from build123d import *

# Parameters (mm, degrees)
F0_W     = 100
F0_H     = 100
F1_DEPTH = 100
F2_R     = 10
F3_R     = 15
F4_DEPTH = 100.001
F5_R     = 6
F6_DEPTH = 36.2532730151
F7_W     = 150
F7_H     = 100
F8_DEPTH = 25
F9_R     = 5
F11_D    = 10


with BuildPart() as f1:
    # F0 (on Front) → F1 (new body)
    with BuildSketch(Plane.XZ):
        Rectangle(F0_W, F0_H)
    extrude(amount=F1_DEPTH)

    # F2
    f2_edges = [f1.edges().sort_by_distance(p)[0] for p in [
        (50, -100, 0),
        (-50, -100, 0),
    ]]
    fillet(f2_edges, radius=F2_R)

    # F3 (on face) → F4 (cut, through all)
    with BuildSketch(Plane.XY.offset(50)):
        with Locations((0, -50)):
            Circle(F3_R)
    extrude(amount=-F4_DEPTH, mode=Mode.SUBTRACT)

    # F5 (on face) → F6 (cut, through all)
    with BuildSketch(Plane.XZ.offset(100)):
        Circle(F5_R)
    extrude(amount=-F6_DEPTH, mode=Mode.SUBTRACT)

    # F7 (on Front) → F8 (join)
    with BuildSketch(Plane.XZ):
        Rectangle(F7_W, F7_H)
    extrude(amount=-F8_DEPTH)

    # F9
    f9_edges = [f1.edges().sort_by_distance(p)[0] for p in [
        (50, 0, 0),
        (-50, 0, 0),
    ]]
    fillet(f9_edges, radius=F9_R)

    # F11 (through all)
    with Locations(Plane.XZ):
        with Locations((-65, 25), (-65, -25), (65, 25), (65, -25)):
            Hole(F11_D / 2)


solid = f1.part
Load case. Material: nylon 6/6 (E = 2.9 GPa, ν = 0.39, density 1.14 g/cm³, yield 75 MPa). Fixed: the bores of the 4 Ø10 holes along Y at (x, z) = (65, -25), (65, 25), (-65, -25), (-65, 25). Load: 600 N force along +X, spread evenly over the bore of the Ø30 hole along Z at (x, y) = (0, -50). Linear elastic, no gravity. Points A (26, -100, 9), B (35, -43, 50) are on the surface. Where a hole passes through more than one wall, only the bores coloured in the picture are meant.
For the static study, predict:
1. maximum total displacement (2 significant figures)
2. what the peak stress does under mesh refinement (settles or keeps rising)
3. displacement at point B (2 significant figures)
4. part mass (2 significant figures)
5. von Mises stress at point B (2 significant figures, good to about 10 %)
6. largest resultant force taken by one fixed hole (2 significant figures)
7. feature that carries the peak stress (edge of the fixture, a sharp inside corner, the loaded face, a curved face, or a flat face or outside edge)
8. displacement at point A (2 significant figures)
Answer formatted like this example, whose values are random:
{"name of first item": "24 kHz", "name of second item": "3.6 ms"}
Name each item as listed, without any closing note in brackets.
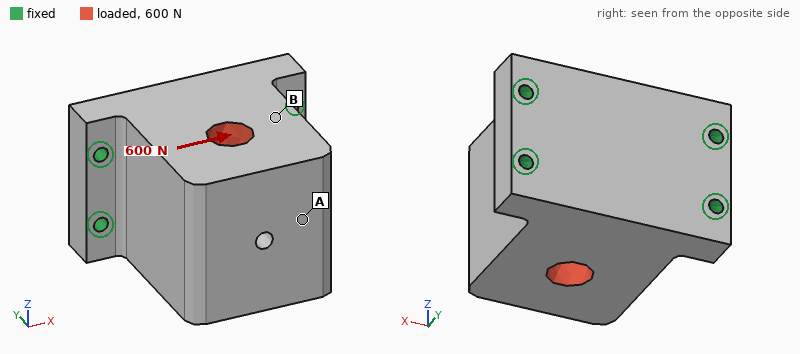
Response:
{"maximum total displacement": "16 µm", "what the peak stress does under mesh refinement": "keeps rising", "displacement at point B": "9.1 µm", "part mass": "1.5 kg", "von Mises stress at point B": "0.13 MPa", "largest resultant force taken by one fixed hole": "220 N", "feature that carries the peak stress": "edge of the fixture", "displacement at point A": "16 µm"}
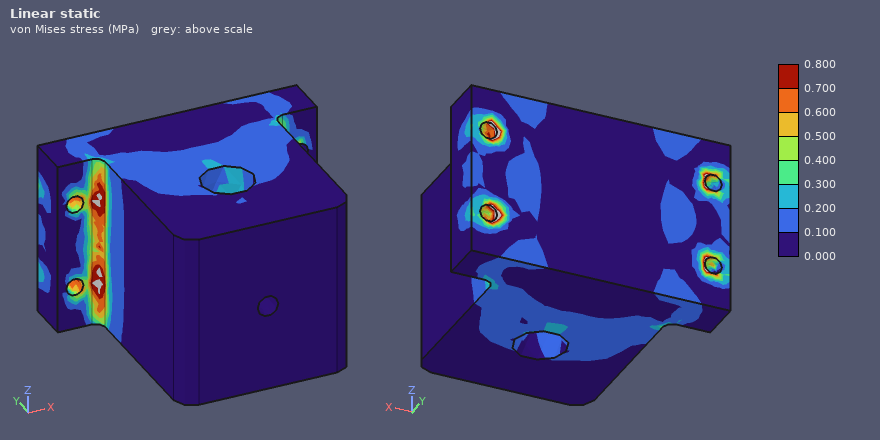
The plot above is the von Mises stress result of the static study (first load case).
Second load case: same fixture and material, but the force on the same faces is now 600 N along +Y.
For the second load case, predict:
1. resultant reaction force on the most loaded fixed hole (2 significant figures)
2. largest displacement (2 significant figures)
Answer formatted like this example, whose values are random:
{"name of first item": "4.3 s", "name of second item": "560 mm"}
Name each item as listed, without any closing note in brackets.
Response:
{"resultant reaction force on the most loaded fixed hole": "160 N", "largest displacement": "7.1 µm"}
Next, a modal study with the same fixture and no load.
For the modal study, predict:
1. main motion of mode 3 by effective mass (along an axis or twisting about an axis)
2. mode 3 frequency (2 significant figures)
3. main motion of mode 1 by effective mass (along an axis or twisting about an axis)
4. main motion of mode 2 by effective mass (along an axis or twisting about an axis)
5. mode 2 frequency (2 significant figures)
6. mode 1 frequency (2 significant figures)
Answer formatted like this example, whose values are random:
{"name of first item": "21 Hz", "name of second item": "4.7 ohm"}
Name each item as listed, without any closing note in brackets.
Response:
{"main motion of mode 3 by effective mass": "along Y", "mode 3 frequency": "1400 Hz", "main motion of mode 1 by effective mass": "along Z", "main motion of mode 2 by effective mass": "along X", "mode 2 frequency": "1100 Hz", "mode 1 frequency": "590 Hz"}
